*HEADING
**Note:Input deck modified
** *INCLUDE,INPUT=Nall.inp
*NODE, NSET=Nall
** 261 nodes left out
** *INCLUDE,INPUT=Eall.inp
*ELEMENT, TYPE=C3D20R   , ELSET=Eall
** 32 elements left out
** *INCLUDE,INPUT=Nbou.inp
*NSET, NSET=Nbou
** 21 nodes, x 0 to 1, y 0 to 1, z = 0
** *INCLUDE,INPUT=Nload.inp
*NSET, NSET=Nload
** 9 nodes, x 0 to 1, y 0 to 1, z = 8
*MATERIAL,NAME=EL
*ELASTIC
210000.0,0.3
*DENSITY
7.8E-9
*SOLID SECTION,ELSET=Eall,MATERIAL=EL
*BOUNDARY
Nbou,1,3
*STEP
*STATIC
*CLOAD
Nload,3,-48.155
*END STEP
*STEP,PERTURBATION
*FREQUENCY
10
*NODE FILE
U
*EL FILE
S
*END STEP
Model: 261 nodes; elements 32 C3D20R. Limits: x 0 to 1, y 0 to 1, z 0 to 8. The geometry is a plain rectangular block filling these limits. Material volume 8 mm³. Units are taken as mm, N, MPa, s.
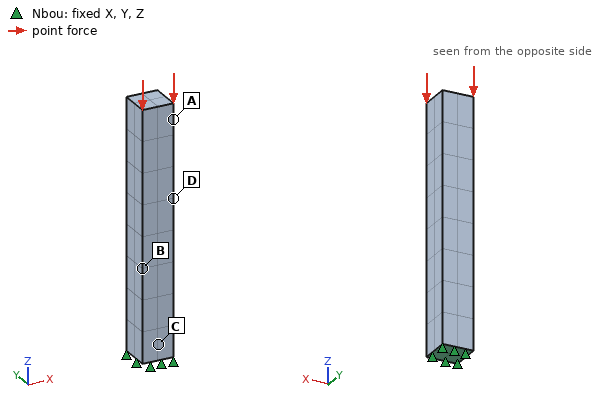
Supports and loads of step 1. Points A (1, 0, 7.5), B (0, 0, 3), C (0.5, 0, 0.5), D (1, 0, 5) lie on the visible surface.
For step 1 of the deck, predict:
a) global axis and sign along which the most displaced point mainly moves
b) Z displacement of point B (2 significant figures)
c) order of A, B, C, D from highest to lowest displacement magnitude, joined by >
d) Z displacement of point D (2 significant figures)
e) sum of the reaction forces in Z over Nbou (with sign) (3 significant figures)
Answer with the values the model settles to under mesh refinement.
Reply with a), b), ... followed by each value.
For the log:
a) -Z
b) -0.0061 mm
c) A > D > B > C
d) -0.010 mm
e) 433 N
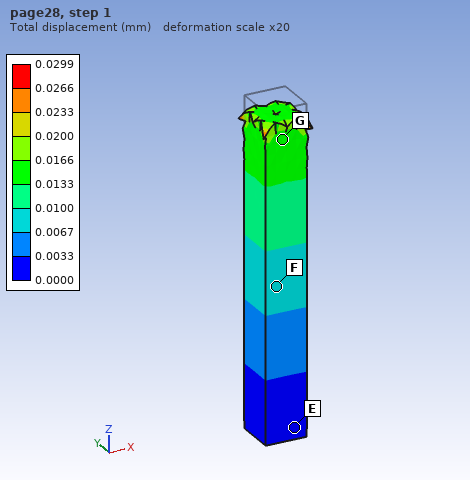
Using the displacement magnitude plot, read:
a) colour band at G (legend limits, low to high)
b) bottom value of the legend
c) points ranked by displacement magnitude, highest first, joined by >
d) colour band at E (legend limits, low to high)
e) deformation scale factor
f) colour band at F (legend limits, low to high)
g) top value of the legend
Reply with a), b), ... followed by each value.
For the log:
a) 0.0133 to 0.0166 mm
b) 0.0000 mm
c) G > F > E
d) 0.0000 to 0.0033 mm
e) 20
f) 0.0067 to 0.0100 mm
g) 0.0299 mm
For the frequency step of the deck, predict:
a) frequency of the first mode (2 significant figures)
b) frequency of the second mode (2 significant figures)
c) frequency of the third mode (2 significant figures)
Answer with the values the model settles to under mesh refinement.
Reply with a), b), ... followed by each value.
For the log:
a) 8000 Hz
b) 8000 Hz
c) 72000 Hz
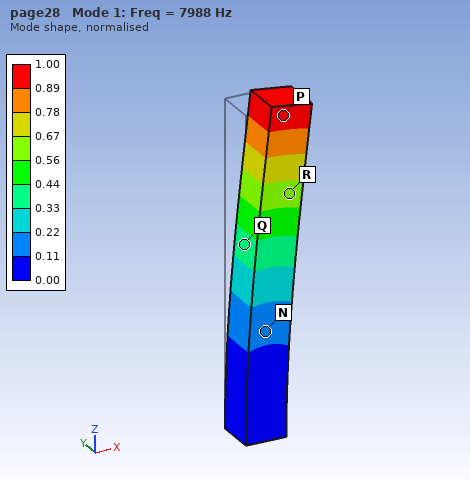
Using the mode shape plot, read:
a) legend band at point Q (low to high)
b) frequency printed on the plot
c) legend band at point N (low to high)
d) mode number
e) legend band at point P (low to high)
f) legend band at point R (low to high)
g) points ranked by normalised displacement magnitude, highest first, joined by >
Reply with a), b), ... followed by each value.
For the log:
a) 0.33 to 0.44
b) 7988 Hz
c) 0.11 to 0.22
d) 1
e) 0.89 to 1.00
f) 0.56 to 0.67
g) P > R > Q > N
